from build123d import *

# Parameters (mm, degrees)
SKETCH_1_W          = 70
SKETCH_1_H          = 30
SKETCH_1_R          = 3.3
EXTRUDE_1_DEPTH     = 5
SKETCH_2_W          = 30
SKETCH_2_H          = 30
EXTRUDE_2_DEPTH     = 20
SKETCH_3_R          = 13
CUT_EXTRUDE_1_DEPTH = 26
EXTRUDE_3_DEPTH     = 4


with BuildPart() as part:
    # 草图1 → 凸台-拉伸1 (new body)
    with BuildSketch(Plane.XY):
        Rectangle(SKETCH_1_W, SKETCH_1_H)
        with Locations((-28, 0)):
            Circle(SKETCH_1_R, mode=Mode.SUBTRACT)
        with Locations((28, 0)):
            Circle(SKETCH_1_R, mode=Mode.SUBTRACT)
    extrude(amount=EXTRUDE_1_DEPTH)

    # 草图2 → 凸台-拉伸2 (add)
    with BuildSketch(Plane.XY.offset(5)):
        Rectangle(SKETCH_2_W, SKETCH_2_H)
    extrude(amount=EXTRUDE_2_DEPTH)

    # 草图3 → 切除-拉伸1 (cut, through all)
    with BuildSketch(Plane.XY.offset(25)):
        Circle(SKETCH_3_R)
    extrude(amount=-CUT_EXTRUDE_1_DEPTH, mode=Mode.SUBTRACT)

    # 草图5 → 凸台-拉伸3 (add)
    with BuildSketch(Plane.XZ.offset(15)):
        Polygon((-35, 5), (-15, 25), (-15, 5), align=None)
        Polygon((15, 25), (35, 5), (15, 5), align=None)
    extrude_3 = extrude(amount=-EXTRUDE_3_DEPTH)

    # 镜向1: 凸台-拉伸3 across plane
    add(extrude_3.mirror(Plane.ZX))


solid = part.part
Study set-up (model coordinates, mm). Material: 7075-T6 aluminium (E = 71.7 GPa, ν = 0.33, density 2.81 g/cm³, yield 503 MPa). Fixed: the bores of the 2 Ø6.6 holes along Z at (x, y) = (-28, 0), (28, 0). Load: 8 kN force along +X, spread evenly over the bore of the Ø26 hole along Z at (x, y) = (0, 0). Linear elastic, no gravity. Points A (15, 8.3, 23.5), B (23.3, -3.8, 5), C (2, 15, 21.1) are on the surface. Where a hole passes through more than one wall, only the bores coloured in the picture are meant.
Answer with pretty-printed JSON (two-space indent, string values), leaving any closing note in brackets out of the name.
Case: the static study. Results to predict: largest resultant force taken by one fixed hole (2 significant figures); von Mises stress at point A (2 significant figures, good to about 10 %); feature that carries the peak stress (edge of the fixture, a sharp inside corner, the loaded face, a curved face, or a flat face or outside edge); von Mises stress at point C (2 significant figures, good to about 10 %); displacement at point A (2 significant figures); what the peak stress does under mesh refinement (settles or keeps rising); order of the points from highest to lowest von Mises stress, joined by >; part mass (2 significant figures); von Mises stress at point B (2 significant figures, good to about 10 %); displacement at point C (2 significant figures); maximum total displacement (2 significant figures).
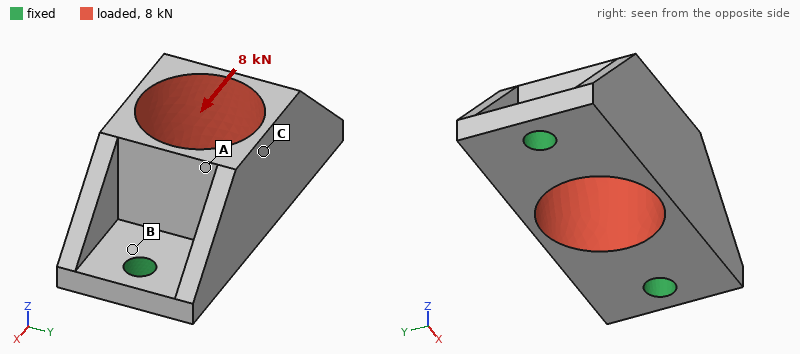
{
  "largest resultant force taken by one fixed hole": "4.3 kN",
  "von Mises stress at point A": "14 MPa",
  "feature that carries the peak stress": "edge of the fixture",
  "von Mises stress at point C": "34 MPa",
  "displacement at point A": "32 µm",
  "what the peak stress does under mesh refinement": "keeps rising",
  "order of the points from highest to lowest von Mises stress, joined by >": "B > C > A",
  "part mass": "51 g",
  "von Mises stress at point B": "53 MPa",
  "displacement at point C": "26 µm",
  "maximum total displacement": "46 µm"
}
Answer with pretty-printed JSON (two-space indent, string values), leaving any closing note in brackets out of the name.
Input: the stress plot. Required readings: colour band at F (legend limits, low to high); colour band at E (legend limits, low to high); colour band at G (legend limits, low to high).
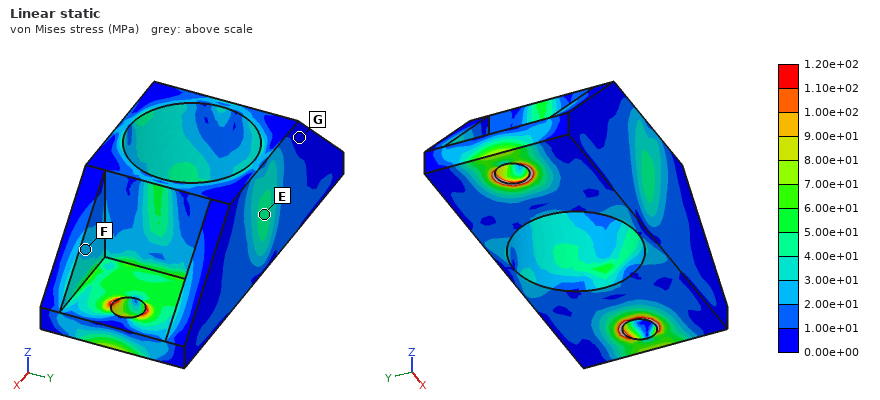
{
  "colour band at F": "2.00e+01 to 3.00e+01 MPa",
  "colour band at E": "4.00e+01 to 5.00e+01 MPa",
  "colour band at G": "0.00e+00 to 1.00e+01 MPa"
}
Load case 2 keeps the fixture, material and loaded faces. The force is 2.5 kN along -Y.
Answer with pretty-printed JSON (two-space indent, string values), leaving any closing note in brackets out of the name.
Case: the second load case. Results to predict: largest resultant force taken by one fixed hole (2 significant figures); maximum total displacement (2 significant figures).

{
  "largest resultant force taken by one fixed hole": "1.3 kN",
  "maximum total displacement": "89 µm"
}
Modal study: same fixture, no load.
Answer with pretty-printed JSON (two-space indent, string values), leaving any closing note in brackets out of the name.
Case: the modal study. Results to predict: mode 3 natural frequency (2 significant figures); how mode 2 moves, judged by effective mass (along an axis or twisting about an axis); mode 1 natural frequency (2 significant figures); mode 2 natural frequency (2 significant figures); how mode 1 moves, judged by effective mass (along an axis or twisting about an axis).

{
  "mode 3 natural frequency": "11 kHz",
  "how mode 2 moves, judged by effective mass": "along Z",
  "mode 1 natural frequency": "5000 Hz",
  "mode 2 natural frequency": "9900 Hz",
  "how mode 1 moves, judged by effective mass": "along Y"
}
